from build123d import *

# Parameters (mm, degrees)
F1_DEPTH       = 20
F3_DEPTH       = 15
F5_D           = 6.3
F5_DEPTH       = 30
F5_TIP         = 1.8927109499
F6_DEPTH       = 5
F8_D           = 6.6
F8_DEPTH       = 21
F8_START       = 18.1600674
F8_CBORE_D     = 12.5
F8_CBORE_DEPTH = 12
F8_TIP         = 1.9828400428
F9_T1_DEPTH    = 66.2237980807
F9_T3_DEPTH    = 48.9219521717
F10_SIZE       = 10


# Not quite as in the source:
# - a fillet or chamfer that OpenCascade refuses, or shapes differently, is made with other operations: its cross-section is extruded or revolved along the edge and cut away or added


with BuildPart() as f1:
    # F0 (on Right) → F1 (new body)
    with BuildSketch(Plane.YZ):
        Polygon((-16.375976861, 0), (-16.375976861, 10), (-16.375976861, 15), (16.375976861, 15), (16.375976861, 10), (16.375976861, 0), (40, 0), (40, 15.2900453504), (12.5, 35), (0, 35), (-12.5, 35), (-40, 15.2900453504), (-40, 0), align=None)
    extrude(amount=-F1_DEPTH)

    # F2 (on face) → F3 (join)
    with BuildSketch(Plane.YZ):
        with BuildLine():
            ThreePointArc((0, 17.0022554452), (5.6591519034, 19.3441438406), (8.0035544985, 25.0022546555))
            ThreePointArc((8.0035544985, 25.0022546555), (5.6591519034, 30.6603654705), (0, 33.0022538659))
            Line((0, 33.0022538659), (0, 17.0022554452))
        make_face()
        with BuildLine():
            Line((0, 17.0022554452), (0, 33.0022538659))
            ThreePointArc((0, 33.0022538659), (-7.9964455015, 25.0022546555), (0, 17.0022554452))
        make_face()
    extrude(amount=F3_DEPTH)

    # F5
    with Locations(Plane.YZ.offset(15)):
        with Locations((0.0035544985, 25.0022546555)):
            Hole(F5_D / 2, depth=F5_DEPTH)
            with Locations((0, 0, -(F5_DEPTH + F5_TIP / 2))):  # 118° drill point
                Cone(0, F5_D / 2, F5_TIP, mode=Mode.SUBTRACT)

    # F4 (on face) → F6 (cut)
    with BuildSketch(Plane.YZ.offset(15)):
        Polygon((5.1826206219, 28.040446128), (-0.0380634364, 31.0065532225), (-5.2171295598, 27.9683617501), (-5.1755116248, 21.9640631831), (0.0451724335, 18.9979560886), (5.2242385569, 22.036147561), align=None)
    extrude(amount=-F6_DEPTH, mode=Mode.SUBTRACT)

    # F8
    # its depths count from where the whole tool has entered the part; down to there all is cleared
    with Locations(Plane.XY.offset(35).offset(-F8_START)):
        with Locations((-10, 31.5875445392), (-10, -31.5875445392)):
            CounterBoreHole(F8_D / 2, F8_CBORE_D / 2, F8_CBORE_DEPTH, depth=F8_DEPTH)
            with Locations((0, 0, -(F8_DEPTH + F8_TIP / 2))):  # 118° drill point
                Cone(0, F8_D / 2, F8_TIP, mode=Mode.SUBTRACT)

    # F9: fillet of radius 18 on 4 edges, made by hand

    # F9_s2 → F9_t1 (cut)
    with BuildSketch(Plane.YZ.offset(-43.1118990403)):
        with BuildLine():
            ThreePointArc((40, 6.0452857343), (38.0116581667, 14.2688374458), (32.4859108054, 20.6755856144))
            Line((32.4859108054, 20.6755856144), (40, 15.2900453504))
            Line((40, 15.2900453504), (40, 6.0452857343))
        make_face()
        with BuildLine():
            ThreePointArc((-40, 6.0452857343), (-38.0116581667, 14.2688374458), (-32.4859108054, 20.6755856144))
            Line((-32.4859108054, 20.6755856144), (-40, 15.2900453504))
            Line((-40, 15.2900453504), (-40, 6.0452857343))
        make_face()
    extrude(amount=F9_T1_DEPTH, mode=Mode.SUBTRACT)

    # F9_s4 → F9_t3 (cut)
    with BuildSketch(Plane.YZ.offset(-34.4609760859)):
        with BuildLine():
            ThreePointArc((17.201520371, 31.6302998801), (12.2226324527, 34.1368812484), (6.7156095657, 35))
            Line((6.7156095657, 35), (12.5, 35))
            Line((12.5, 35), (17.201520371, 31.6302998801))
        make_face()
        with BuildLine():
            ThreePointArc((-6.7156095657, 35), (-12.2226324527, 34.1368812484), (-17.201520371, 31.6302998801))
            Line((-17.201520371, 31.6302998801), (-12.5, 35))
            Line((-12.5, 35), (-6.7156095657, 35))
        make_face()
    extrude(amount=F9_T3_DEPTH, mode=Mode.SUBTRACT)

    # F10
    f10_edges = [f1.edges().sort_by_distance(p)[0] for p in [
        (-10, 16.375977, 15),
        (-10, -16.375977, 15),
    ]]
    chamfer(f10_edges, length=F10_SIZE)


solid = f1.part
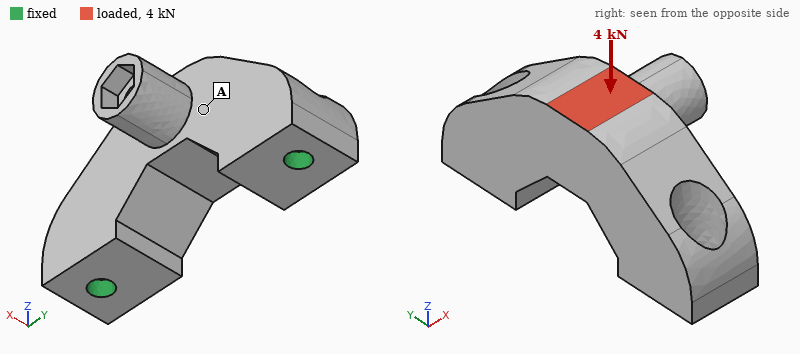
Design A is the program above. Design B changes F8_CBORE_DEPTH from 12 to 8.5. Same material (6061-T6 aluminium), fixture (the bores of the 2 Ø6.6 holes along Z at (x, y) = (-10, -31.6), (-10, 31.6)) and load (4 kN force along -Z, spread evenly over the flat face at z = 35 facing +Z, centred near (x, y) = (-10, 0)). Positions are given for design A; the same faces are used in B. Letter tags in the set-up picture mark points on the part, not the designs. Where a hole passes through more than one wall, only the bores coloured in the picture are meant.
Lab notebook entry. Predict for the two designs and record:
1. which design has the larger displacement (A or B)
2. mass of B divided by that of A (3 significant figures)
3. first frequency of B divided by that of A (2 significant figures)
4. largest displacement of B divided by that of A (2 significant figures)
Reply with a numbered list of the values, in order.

1. A
2. 1.02
3. 1.5
4. 0.82
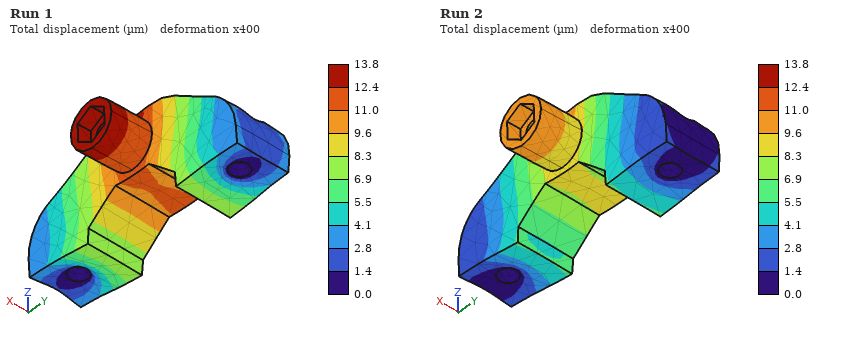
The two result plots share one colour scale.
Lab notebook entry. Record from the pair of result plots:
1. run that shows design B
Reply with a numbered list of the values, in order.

1. Run 2
